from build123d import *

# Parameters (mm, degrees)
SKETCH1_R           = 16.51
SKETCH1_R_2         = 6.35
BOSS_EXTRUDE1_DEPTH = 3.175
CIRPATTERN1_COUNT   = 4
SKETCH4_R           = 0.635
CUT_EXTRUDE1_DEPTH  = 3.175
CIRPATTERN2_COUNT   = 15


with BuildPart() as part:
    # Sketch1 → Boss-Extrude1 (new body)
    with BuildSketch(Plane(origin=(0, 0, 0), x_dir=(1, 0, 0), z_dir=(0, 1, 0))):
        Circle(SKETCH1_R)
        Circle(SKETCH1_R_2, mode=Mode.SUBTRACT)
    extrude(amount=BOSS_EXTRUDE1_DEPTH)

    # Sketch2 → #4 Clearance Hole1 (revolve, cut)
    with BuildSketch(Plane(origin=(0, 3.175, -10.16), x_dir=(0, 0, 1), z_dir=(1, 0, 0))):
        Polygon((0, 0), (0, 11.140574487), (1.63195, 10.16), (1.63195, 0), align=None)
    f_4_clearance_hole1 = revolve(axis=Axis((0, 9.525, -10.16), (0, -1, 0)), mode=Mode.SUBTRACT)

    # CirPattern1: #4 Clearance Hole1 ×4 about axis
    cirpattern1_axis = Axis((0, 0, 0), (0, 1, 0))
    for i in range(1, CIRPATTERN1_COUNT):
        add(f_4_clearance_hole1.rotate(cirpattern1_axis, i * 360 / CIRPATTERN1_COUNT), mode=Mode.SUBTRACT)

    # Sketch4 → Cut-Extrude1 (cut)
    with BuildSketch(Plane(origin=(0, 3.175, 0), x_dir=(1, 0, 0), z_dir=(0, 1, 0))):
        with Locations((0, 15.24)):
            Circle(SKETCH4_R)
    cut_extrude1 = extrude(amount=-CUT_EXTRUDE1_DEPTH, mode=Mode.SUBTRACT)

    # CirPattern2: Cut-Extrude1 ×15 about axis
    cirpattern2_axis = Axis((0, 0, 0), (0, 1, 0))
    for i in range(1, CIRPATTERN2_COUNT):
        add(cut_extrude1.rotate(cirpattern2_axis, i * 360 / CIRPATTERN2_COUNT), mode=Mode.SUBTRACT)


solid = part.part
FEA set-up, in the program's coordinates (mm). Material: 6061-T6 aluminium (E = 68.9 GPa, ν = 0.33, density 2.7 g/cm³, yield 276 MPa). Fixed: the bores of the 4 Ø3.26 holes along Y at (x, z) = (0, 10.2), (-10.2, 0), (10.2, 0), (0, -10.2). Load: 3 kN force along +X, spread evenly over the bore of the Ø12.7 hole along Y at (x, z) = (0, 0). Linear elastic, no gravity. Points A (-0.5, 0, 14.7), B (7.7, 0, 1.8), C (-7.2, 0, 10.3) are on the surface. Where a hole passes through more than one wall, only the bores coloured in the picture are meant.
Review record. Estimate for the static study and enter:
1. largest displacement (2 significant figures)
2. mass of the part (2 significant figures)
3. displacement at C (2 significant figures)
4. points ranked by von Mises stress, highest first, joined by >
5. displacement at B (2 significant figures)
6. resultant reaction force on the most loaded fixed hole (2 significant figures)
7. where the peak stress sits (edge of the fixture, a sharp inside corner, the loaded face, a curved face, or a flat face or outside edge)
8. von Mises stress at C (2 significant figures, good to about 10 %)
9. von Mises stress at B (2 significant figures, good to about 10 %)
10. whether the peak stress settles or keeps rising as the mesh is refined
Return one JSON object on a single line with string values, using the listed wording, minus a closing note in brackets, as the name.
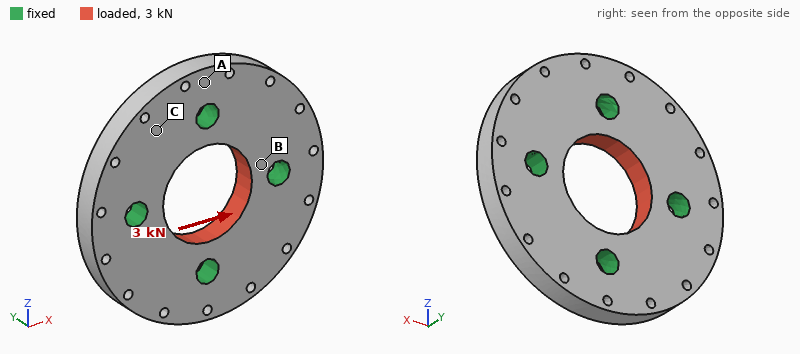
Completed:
{"largest displacement": "3.0 µm", "mass of the part": "5.8 g", "displacement at C": "1.3 µm", "points ranked by von Mises stress, highest first, joined by >": "B > C > A", "displacement at B": "1.1 µm", "resultant reaction force on the most loaded fixed hole": "770 N", "where the peak stress sits": "edge of the fixture", "von Mises stress at C": "9.0 MPa", "von Mises stress at B": "33 MPa", "whether the peak stress settles or keeps rising as the mesh is refined": "keeps rising"}
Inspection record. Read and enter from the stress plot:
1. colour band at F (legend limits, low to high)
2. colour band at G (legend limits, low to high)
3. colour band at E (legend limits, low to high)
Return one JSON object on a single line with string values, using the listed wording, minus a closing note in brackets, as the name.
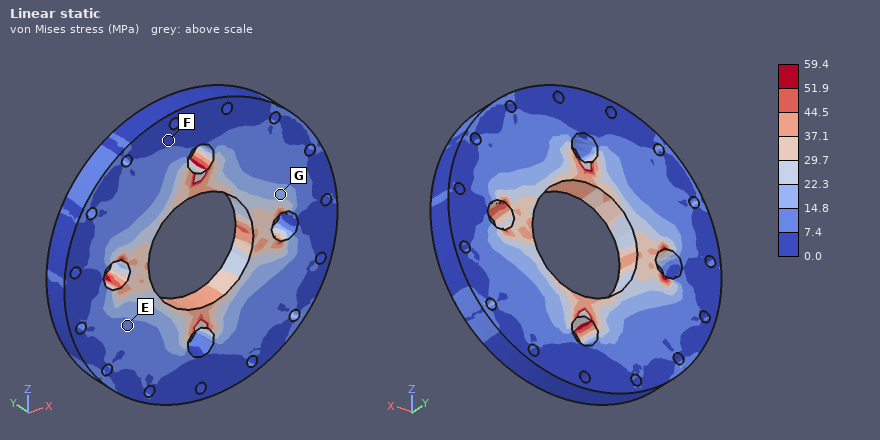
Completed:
{"colour band at F": "0.0 to 7.4 MPa", "colour band at G": "14.8 to 22.3 MPa", "colour band at E": "7.4 to 14.8 MPa"}
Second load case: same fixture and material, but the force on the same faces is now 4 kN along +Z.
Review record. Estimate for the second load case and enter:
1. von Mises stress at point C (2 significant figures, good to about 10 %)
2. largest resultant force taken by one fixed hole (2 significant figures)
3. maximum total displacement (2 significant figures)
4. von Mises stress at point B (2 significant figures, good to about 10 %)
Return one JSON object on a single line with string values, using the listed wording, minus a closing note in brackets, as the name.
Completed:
{"von Mises stress at point C": "11 MPa", "largest resultant force taken by one fixed hole": "1.0 kN", "maximum total displacement": "4.0 µm", "von Mises stress at point B": "38 MPa"}
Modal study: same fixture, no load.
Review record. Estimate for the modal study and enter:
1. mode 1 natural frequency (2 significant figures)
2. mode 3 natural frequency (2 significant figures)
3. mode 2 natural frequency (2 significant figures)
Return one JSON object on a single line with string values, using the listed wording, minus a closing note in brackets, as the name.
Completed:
{"mode 1 natural frequency": "32 kHz", "mode 3 natural frequency": "34 kHz", "mode 2 natural frequency": "34 kHz"}
